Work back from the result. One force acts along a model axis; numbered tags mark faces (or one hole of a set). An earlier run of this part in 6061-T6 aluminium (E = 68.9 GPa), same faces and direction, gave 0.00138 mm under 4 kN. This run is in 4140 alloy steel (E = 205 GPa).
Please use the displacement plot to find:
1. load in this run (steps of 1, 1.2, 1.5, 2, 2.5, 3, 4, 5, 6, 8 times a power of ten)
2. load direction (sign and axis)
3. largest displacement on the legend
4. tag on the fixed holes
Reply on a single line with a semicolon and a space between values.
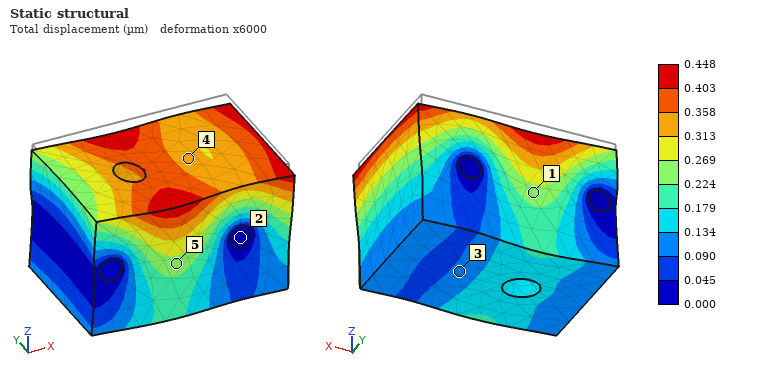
4 kN; -Z; 0.448 µm; 2
